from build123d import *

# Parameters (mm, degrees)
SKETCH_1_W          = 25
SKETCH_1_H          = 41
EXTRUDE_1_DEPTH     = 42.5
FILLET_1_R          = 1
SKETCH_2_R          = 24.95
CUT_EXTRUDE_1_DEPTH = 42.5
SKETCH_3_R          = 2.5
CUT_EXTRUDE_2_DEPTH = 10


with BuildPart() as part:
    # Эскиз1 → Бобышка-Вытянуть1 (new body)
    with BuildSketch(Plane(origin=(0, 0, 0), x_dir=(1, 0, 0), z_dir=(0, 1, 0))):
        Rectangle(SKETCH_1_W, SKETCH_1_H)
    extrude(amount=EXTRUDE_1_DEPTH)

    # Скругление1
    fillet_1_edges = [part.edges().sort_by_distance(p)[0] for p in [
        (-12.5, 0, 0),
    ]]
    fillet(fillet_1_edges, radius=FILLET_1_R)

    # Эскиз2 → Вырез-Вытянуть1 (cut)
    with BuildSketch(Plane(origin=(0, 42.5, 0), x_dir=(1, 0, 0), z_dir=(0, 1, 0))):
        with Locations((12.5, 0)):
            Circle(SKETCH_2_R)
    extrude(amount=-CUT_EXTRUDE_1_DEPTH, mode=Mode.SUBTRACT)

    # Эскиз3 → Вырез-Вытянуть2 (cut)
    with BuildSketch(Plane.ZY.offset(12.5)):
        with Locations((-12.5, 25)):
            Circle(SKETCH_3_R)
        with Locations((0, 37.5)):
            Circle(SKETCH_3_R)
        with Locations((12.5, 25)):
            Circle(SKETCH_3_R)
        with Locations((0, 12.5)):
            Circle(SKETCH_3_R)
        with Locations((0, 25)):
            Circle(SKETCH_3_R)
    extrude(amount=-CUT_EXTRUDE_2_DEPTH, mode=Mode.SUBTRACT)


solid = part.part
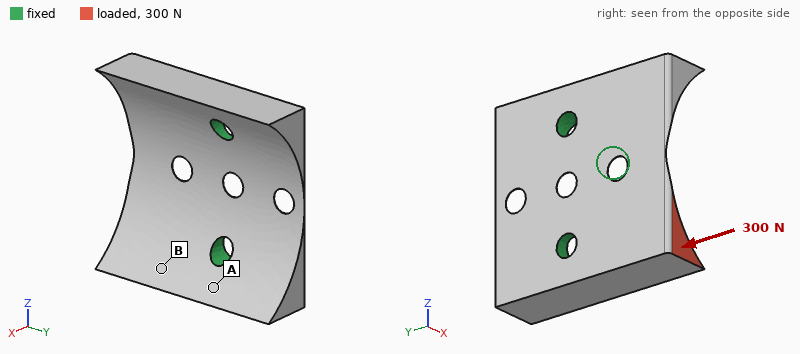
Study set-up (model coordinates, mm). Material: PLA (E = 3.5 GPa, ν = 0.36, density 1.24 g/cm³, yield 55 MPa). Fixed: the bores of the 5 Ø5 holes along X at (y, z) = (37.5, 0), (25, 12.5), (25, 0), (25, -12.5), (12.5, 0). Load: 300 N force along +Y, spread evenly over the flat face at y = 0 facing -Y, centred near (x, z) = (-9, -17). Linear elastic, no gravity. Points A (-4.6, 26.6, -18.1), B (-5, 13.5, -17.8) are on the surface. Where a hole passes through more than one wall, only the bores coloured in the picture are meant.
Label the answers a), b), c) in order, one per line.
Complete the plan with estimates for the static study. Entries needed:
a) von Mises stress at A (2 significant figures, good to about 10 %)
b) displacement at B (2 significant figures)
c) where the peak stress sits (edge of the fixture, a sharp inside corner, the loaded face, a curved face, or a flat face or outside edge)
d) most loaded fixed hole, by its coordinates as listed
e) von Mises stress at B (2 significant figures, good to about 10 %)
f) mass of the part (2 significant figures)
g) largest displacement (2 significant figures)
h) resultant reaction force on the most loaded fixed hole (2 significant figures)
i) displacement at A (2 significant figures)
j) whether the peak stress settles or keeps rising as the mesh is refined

a) 3.0 MPa
b) 0.059 mm
c) edge of the fixture
d) (25, -12.5)
e) 7.3 MPa
f) 6.8 g
g) 0.15 mm
h) 310 N
i) 0.024 mm
j) keeps rising
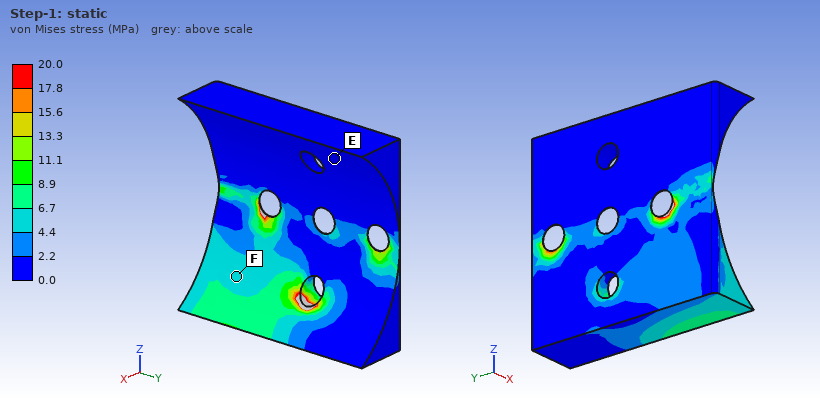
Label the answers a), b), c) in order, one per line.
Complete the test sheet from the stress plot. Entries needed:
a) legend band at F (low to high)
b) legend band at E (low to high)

a) 4.4 to 6.7 MPa
b) 0.0 to 2.2 MPa
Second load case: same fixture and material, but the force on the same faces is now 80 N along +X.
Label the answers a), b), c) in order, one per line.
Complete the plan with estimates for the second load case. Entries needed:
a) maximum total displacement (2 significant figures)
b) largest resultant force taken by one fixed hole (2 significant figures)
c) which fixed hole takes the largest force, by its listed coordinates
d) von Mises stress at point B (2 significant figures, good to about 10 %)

a) 0.72 mm
b) 84 N
c) (25, -12.5)
d) 15 MPa
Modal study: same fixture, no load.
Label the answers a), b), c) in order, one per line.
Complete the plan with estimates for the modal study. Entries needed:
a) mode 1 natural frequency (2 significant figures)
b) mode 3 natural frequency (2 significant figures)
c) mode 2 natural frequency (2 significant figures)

a) 2300 Hz
b) 4800 Hz
c) 2300 Hz
